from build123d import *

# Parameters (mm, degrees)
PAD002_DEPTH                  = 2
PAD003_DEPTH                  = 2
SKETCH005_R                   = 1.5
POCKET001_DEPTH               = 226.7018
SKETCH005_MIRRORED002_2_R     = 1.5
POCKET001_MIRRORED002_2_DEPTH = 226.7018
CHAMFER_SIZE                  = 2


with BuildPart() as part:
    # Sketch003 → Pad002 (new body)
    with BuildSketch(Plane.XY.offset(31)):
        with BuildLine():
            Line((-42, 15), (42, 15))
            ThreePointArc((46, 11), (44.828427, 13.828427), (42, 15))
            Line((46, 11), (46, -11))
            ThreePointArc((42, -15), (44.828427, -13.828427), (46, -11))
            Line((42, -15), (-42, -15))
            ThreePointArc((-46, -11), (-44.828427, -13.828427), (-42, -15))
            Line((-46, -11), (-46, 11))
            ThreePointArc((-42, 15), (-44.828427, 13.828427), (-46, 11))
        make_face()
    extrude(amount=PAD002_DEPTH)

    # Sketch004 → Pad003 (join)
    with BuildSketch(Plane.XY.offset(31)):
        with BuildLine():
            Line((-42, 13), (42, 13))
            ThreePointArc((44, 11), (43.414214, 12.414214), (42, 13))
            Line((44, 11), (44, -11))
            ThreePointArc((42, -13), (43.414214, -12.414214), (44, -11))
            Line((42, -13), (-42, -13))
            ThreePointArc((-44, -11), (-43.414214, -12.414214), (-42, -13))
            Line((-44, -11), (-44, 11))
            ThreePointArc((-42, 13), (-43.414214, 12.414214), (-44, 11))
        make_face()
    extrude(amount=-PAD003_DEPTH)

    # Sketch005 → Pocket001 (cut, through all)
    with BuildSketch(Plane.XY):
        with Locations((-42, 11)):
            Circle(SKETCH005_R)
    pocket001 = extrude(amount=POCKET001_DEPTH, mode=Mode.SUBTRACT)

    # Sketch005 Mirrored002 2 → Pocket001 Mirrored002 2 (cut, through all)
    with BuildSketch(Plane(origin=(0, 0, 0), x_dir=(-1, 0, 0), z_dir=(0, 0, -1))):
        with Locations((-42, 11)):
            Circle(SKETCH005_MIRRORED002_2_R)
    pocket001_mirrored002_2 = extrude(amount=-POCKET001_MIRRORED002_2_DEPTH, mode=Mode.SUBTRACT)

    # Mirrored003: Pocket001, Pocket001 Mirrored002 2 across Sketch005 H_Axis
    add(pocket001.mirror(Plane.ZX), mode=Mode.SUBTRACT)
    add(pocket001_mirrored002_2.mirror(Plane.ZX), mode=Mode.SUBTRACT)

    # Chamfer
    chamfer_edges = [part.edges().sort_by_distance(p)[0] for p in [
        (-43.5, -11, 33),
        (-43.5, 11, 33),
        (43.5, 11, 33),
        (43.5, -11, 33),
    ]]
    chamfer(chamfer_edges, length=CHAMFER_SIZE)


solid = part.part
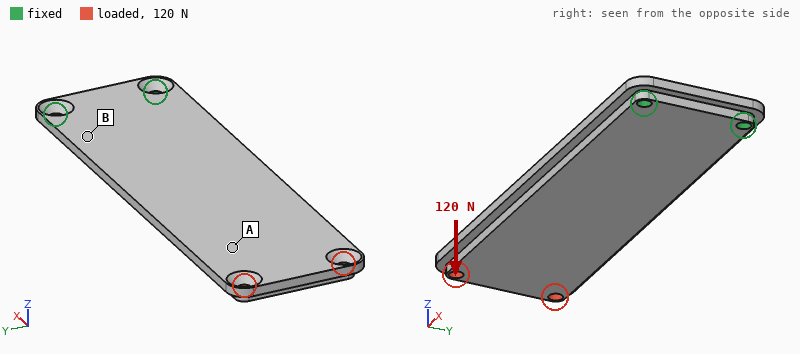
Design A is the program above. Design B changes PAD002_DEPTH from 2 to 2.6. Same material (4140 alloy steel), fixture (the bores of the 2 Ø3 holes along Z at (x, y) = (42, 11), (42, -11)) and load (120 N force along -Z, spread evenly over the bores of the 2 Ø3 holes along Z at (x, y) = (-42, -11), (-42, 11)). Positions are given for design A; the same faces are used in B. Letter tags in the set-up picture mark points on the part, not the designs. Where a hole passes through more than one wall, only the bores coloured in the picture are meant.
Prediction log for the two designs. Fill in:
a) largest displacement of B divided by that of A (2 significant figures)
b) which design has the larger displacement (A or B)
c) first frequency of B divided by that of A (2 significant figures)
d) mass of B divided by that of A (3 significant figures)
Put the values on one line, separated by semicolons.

0.63; A; 1.2; 1.17
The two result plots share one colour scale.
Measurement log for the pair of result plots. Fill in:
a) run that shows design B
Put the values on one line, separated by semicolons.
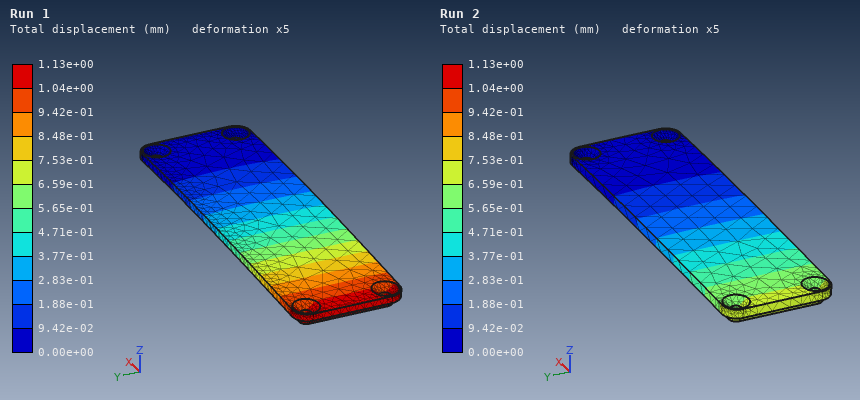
Run 2
